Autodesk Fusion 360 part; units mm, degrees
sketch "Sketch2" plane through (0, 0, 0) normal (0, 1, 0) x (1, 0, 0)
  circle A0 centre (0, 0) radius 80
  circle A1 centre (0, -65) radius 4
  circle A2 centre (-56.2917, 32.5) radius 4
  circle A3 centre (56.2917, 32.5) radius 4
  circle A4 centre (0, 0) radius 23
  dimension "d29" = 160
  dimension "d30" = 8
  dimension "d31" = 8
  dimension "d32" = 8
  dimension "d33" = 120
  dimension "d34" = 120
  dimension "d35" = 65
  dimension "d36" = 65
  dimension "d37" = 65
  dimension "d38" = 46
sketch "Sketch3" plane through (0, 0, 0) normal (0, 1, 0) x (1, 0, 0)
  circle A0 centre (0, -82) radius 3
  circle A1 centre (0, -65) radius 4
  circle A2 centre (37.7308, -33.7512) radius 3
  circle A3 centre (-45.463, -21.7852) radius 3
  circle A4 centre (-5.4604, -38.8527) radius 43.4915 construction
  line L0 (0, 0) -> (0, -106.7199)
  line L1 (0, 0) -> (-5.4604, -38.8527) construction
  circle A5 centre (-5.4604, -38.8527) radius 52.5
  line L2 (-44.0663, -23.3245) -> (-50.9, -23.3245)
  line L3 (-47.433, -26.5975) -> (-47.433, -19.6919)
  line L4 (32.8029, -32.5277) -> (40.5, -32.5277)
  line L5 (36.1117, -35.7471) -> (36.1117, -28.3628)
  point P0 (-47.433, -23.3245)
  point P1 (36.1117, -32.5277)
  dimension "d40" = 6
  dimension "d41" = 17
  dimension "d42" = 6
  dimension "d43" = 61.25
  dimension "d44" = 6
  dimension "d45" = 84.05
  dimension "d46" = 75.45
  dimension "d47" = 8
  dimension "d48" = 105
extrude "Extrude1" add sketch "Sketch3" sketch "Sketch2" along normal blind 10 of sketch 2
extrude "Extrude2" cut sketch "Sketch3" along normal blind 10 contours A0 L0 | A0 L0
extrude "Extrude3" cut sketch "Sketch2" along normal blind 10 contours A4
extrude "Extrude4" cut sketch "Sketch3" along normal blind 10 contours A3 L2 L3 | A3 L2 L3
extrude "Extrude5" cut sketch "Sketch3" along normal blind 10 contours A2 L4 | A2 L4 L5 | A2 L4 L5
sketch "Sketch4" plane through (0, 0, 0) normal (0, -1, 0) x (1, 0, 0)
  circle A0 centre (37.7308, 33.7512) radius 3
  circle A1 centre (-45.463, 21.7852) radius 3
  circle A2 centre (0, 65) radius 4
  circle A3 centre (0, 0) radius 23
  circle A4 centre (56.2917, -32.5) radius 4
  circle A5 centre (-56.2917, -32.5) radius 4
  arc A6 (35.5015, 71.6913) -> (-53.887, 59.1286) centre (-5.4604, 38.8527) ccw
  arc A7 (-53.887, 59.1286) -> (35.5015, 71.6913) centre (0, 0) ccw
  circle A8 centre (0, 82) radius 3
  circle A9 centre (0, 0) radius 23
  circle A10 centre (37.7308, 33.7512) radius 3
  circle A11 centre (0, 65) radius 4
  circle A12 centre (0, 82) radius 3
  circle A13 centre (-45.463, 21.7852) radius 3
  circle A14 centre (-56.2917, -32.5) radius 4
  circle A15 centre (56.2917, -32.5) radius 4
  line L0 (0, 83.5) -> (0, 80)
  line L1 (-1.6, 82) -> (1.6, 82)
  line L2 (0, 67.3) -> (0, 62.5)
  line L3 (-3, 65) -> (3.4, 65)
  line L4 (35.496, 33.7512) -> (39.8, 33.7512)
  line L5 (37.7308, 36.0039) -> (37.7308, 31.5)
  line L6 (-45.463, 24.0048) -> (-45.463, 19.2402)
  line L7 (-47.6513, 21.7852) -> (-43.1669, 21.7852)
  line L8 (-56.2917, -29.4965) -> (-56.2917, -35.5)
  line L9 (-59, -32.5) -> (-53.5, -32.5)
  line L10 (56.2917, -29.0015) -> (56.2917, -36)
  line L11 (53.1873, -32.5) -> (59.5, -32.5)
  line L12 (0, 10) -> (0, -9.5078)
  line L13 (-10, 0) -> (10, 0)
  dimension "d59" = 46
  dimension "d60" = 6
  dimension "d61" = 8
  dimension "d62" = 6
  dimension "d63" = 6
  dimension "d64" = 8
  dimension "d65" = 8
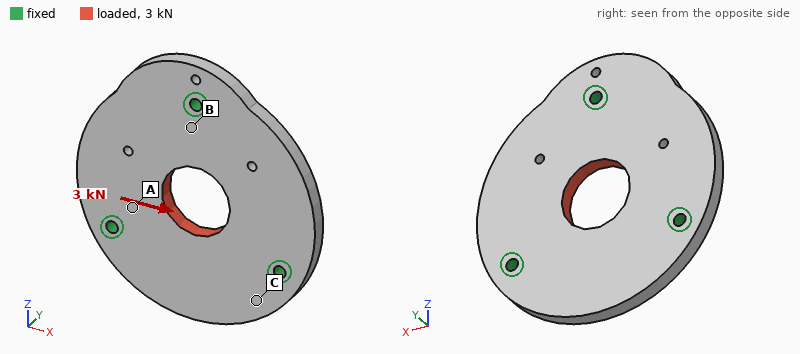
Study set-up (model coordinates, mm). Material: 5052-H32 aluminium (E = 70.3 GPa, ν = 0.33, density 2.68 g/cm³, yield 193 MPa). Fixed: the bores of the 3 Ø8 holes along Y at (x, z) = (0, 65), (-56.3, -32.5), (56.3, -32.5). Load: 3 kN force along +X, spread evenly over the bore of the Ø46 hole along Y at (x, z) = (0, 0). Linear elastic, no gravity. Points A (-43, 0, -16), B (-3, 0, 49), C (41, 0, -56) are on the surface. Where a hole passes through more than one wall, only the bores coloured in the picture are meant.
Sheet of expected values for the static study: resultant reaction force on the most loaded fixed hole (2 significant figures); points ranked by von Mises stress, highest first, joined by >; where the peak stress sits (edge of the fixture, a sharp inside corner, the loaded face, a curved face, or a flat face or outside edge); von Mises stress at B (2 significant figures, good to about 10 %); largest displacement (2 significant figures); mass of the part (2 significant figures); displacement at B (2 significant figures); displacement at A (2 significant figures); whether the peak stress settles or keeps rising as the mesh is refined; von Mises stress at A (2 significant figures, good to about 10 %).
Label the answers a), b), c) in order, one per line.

a) 1.0 kN
b) A > B > C
c) edge of the fixture
d) 1.3 MPa
e) 3.1 µm
f) 510 g
g) 1.2 µm
h) 1.4 µm
i) keeps rising
j) 2.5 MPa
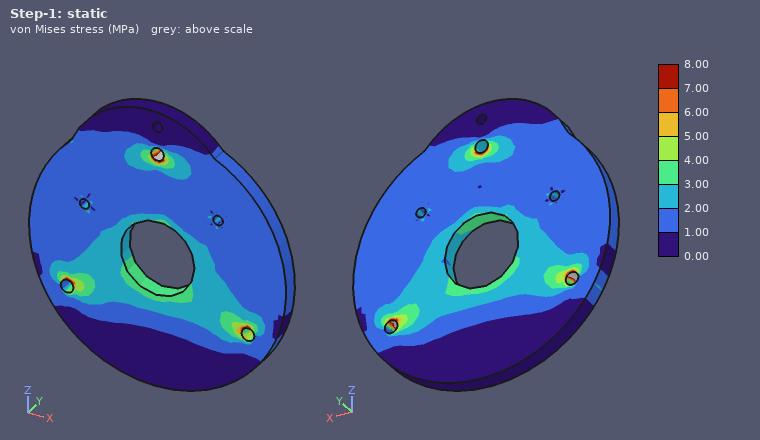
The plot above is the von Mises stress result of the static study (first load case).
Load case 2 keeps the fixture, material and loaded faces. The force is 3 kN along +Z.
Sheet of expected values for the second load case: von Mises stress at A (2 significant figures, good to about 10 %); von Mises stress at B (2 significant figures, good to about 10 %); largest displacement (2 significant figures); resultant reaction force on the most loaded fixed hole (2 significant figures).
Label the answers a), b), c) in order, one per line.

a) 1.9 MPa
b) 3.5 MPa
c) 3.3 µm
d) 1.0 kN
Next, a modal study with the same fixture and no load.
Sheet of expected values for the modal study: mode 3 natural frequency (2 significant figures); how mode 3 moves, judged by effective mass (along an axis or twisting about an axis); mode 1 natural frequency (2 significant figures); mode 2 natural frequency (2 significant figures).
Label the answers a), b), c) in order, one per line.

a) 2900 Hz
b) along Y
c) 2500 Hz
d) 2500 Hz
